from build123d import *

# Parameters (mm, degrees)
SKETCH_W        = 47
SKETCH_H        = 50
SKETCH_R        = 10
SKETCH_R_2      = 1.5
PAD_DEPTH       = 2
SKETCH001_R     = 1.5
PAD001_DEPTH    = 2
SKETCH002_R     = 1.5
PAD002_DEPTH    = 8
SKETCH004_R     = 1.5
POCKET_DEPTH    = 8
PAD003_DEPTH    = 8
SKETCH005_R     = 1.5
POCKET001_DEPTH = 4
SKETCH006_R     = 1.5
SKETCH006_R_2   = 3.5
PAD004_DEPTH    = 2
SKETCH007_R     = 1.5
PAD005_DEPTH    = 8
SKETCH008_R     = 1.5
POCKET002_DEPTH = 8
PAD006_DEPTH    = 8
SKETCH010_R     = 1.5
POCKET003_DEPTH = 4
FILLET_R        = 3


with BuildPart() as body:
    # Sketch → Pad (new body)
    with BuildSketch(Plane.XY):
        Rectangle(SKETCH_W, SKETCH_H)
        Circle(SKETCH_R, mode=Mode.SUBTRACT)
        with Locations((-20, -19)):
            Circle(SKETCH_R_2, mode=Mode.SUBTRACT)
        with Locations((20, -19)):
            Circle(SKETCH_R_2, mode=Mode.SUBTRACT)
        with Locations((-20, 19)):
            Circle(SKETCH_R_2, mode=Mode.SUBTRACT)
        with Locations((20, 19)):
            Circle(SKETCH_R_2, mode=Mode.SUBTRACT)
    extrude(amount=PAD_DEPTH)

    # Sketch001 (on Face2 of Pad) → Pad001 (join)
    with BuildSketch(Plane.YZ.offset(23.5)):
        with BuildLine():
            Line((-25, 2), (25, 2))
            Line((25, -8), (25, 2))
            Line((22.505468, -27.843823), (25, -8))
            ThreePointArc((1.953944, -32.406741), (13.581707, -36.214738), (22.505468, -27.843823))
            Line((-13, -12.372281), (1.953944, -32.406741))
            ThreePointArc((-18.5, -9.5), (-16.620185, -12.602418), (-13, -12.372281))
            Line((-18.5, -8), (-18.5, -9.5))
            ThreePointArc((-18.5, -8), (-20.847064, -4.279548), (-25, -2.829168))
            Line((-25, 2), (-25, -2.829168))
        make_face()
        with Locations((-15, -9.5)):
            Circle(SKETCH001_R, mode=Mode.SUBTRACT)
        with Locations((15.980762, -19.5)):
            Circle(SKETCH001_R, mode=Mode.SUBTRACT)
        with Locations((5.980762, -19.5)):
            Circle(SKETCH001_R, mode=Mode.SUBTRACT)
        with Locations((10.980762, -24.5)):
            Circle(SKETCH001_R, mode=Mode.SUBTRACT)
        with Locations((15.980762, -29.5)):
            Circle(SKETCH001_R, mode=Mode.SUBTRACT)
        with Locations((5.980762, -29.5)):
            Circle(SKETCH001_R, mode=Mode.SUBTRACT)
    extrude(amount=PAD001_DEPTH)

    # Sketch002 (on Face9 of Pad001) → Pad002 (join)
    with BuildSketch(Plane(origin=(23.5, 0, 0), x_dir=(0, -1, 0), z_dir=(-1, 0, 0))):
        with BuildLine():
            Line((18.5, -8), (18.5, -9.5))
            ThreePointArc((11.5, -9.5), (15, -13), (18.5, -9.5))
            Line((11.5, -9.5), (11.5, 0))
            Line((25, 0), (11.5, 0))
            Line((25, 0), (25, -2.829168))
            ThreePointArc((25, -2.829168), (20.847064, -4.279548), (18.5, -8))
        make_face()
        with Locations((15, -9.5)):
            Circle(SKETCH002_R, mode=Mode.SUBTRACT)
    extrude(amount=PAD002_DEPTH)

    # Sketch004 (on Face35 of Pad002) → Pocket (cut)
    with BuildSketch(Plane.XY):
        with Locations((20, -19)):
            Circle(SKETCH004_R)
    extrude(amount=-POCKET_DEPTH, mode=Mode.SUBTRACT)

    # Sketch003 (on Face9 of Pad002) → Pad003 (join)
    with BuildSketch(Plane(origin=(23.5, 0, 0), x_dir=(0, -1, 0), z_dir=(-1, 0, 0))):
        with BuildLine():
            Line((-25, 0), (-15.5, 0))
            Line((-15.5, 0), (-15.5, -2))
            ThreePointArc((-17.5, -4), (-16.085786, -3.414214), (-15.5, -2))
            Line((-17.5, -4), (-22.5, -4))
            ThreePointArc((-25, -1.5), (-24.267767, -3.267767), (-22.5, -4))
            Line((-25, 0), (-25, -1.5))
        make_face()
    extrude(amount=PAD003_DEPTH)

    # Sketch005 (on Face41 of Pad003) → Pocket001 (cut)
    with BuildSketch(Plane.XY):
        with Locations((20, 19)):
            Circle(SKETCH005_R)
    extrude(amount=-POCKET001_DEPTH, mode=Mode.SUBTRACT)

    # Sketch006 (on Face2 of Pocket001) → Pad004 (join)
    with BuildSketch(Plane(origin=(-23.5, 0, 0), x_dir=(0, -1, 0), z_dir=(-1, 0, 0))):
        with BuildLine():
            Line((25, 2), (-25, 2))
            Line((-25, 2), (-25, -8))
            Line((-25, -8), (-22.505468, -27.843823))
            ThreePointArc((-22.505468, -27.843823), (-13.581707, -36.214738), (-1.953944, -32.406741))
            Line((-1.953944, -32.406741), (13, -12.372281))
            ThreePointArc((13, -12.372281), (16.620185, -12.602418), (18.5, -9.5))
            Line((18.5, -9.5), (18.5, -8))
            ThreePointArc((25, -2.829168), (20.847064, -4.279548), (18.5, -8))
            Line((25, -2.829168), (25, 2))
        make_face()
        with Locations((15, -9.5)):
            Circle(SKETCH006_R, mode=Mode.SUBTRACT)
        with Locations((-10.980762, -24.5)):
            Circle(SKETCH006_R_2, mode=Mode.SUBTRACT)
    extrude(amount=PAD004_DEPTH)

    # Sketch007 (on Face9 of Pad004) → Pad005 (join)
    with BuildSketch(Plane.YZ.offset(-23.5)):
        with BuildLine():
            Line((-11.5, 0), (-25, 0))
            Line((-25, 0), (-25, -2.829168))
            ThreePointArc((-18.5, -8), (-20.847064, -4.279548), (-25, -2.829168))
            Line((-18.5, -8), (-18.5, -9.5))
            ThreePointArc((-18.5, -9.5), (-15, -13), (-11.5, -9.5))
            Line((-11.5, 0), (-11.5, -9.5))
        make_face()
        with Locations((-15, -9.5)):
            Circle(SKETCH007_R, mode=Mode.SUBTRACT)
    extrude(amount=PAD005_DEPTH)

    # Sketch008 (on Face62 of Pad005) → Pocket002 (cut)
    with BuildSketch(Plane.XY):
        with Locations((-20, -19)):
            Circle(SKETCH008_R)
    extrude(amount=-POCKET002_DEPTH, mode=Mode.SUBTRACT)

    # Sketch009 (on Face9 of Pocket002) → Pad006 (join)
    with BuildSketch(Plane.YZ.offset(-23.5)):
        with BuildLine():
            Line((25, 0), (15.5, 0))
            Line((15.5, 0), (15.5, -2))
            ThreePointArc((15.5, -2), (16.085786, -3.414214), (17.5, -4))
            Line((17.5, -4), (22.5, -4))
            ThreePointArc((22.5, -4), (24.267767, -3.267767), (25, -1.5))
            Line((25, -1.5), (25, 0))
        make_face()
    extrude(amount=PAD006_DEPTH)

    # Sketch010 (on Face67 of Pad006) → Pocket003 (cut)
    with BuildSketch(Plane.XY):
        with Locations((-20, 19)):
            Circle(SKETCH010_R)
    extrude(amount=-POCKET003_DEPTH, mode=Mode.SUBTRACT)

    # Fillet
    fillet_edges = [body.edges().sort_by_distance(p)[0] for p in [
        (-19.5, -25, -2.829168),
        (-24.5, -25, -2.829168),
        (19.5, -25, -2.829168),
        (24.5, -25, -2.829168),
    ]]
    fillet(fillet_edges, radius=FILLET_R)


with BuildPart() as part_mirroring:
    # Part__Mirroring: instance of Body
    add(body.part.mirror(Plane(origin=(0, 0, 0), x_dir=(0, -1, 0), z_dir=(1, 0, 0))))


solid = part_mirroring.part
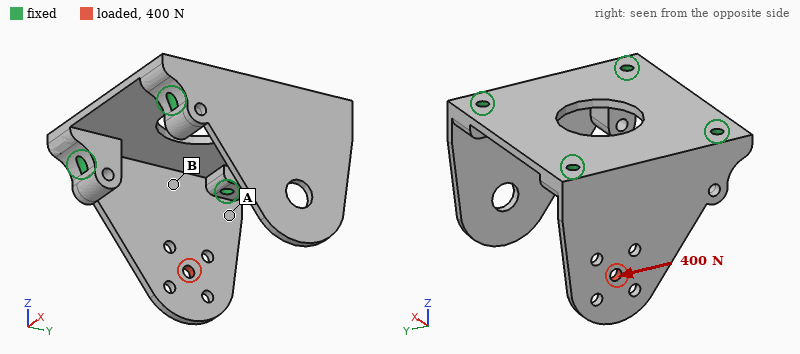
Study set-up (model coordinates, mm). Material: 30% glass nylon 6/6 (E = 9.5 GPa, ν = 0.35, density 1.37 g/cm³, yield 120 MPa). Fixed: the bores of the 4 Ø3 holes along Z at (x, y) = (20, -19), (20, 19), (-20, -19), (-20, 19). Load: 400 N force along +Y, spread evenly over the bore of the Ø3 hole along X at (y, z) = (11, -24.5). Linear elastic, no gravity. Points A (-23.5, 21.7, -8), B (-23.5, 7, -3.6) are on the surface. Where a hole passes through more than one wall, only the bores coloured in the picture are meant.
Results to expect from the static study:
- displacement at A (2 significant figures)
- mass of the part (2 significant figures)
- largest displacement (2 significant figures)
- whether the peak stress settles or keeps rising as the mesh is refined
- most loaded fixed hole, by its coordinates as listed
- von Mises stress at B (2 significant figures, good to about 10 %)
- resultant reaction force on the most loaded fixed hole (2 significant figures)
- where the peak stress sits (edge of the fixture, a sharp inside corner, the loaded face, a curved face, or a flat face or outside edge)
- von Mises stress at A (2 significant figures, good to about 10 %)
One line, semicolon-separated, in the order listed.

29 µm; 15 g; 99 µm; keeps rising; (-20, -19); 4.7 MPa; 350 N; edge of the fixture; 14 MPa
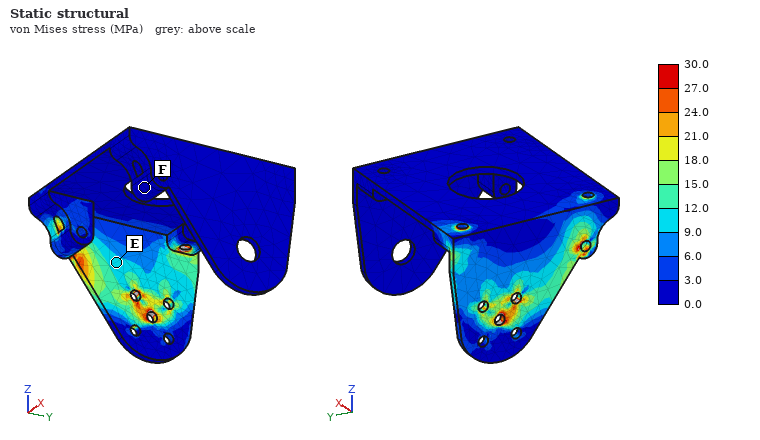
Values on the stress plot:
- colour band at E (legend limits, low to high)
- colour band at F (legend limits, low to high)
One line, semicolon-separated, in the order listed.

9.0 to 12.0 MPa; 0.0 to 3.0 MPa
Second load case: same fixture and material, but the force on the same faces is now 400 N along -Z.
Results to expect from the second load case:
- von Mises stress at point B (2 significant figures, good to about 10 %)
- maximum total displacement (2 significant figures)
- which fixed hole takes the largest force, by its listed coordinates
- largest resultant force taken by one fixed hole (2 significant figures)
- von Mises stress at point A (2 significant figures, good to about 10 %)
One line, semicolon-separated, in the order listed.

2.7 MPa; 84 µm; (-20, 19); 300 N; 11 MPa
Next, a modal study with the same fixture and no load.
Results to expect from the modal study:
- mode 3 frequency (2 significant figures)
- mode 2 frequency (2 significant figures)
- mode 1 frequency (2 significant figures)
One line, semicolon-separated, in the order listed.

3300 Hz; 1000 Hz; 1000 Hz
